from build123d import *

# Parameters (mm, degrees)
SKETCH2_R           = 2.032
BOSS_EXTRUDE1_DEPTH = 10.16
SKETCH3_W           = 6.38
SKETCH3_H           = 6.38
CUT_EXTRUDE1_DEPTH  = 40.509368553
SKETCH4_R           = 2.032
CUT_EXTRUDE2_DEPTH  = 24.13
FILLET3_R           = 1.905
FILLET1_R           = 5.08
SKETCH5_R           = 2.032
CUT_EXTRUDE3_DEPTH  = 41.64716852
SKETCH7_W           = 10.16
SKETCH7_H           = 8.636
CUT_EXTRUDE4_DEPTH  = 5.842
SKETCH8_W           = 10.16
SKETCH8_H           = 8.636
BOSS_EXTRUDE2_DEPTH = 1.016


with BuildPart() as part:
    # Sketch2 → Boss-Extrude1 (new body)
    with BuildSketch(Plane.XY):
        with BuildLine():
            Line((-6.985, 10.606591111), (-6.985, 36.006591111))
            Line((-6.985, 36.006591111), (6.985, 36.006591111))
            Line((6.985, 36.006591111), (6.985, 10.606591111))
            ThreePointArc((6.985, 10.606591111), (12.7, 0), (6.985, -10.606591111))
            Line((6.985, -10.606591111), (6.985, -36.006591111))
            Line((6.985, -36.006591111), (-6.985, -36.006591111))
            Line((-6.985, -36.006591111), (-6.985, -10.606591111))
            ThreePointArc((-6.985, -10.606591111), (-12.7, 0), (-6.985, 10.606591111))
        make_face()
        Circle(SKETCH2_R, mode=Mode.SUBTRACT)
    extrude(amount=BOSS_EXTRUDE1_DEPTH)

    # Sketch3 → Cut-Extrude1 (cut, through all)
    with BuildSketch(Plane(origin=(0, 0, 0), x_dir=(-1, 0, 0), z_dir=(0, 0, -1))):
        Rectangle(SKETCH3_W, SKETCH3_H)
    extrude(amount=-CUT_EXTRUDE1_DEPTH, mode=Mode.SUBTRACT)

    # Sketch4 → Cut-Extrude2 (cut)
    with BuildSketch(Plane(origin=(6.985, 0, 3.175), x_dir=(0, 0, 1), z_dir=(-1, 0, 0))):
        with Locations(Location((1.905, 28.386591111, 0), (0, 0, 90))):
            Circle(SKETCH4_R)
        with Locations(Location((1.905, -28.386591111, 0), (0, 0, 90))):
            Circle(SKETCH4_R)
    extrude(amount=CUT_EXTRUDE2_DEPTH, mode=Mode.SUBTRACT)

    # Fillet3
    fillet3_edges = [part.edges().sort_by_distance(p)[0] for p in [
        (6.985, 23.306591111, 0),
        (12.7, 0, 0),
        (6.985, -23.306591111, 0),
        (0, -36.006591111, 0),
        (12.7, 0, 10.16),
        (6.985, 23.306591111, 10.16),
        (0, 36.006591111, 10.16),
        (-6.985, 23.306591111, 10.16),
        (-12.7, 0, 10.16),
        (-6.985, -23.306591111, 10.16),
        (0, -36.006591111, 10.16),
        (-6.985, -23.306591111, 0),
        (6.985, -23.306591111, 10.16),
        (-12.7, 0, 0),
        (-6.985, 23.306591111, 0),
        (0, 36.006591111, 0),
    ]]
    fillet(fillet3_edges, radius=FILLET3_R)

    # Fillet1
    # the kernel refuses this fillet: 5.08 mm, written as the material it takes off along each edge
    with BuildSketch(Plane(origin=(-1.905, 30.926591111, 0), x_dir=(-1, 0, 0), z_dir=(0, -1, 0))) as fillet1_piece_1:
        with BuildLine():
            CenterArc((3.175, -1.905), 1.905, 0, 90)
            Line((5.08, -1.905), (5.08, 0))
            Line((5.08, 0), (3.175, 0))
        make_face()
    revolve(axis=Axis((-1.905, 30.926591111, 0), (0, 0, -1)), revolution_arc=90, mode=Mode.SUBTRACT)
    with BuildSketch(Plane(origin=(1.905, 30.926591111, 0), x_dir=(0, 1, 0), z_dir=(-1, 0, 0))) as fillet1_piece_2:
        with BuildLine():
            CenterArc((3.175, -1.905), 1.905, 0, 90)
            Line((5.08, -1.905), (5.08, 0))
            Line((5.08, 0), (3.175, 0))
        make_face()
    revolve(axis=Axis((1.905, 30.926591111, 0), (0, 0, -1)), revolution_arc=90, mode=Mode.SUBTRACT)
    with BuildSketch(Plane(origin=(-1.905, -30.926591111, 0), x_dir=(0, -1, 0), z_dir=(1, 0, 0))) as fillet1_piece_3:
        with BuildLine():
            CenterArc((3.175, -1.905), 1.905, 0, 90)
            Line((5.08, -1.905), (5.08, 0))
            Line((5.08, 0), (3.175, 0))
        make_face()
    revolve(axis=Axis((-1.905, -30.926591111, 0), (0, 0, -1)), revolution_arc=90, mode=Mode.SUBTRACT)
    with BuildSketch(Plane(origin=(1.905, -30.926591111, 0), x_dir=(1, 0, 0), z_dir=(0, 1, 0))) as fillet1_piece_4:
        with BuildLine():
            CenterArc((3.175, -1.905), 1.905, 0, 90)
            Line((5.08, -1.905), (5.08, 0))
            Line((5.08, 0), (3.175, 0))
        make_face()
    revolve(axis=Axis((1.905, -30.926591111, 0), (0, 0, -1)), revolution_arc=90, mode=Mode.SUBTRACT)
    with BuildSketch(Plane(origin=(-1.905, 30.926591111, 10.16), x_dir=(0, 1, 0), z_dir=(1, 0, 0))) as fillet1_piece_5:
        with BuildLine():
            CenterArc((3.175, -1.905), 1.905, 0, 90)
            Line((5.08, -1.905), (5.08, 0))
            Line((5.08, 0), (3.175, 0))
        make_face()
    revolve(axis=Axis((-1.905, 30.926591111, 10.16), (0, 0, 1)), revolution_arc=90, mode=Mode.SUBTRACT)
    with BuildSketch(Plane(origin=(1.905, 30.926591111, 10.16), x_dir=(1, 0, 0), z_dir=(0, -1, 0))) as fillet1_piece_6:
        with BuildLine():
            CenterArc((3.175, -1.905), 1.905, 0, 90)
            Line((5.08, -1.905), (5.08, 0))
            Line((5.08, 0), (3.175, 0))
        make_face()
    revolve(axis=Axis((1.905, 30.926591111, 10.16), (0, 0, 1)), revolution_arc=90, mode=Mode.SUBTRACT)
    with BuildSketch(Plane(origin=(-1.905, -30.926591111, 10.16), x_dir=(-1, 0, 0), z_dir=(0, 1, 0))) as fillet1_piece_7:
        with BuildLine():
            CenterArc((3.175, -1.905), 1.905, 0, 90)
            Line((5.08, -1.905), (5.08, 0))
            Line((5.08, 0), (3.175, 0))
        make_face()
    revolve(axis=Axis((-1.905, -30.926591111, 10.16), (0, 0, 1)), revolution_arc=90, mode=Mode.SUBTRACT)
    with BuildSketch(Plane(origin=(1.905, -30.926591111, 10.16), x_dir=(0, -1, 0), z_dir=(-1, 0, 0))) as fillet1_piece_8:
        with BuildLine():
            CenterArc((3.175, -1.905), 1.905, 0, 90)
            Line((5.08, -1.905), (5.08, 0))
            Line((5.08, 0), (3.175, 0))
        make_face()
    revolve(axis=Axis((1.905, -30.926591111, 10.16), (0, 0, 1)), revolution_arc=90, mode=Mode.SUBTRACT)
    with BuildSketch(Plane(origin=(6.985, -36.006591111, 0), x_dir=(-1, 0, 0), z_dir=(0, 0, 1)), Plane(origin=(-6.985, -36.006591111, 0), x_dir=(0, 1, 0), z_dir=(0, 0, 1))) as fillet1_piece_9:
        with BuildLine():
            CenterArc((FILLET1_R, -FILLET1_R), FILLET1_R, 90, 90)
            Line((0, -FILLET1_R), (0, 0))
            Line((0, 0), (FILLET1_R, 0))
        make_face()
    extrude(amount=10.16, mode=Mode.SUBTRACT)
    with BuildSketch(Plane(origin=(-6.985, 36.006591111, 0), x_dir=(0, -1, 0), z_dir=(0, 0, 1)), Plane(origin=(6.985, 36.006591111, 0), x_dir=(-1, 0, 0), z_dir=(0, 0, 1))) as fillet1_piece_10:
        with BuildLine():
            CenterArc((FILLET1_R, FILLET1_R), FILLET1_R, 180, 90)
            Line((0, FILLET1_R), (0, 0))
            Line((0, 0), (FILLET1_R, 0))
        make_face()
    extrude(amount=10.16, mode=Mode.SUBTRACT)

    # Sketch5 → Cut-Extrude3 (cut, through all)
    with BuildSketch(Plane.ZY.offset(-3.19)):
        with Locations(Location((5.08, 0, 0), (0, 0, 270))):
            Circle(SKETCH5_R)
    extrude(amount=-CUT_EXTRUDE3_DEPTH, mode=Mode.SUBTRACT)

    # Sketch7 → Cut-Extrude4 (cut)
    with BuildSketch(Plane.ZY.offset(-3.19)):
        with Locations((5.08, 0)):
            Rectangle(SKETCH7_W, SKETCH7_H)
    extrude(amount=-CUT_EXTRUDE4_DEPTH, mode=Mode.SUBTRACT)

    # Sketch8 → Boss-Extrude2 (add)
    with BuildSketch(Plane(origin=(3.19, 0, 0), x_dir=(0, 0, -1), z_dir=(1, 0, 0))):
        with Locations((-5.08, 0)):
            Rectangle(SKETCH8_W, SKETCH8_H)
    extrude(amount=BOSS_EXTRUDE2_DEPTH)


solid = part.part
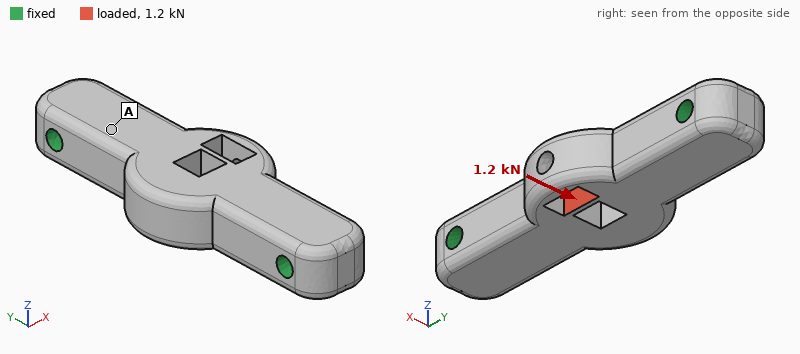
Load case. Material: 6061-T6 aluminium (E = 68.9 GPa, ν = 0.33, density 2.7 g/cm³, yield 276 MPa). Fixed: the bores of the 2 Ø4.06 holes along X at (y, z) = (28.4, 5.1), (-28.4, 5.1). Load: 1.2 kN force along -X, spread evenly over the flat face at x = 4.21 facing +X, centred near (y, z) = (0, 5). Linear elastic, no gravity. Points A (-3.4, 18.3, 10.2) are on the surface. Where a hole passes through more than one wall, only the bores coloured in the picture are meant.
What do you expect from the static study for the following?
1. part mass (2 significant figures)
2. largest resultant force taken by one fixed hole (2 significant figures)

28 g
600 N
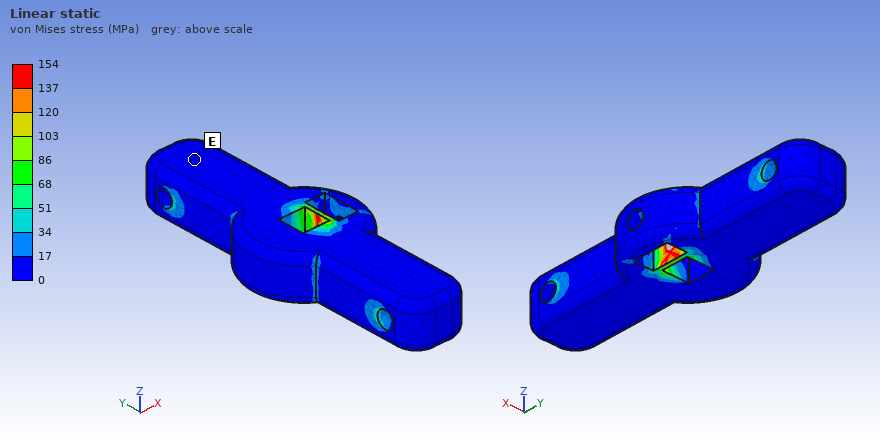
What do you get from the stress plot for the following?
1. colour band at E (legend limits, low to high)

0 to 17 MPa
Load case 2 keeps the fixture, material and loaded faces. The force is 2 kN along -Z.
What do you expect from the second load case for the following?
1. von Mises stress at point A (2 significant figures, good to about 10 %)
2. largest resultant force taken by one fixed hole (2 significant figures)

25 MPa
1.0 kN
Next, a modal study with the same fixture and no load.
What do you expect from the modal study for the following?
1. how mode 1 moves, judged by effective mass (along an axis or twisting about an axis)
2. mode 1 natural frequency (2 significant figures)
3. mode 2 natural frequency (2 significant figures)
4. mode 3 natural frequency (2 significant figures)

along Z
11 kHz
17 kHz
17 kHz
